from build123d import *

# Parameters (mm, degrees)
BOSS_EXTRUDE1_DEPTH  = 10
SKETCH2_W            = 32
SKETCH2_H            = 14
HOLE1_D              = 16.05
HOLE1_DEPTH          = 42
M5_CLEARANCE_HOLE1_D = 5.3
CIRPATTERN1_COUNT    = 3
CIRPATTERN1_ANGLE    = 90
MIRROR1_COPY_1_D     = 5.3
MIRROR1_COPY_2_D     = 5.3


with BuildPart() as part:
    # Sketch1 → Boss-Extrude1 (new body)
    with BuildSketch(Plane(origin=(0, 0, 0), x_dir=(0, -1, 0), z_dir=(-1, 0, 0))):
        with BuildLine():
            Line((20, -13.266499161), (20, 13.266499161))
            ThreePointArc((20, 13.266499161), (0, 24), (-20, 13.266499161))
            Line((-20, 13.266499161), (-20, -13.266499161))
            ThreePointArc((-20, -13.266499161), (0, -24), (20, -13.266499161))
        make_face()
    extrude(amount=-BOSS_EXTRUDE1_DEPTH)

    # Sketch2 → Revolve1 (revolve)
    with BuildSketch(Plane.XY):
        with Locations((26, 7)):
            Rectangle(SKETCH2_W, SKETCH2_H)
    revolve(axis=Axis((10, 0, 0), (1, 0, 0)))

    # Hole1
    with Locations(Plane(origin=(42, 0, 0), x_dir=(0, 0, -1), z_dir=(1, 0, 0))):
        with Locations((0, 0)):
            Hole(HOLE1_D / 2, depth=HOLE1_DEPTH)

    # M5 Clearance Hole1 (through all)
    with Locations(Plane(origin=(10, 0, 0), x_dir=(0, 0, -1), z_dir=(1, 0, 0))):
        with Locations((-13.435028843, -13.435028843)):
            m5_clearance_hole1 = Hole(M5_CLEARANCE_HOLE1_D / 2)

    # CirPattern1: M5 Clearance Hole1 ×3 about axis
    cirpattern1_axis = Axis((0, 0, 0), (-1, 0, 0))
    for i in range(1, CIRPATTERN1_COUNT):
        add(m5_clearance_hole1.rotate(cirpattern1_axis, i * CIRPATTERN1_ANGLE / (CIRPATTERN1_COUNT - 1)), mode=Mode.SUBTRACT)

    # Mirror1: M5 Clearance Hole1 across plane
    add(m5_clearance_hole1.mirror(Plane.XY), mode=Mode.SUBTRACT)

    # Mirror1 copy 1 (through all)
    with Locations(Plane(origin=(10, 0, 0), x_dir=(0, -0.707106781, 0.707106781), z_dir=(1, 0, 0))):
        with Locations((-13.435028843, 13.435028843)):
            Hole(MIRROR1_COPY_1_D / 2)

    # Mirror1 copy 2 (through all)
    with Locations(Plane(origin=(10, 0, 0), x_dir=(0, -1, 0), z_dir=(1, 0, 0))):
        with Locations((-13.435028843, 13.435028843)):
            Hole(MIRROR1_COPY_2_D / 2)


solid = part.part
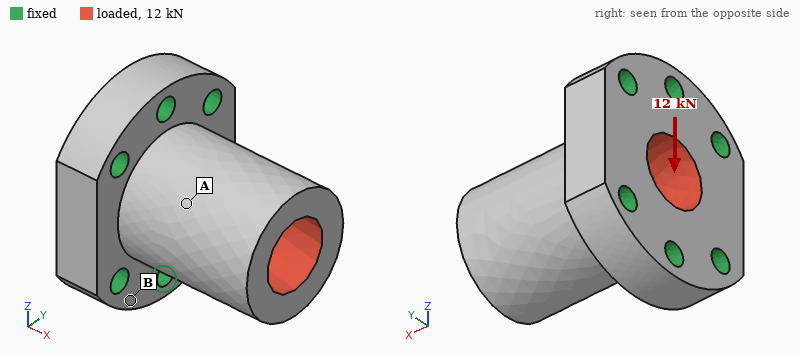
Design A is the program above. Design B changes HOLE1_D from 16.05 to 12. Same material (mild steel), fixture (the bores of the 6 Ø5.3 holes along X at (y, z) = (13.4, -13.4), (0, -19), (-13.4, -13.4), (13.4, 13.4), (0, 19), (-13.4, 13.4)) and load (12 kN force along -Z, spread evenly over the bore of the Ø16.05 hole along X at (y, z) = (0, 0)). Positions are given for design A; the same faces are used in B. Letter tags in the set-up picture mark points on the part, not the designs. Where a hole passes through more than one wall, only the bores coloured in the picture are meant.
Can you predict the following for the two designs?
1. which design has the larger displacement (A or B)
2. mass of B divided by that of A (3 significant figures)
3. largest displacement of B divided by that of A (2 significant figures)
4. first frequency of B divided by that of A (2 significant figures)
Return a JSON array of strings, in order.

["A", "1.14", "0.87", "0.97"]
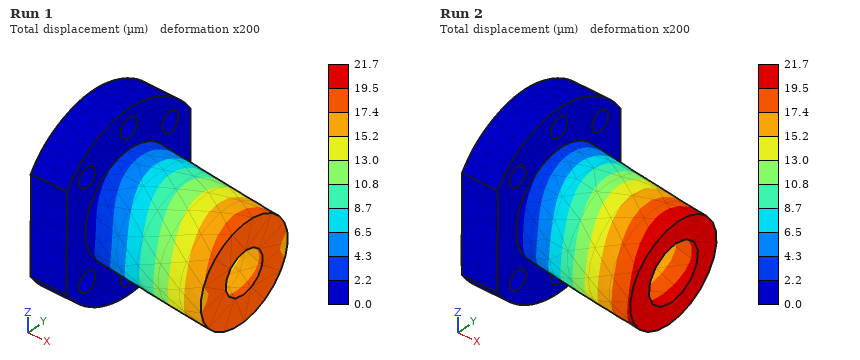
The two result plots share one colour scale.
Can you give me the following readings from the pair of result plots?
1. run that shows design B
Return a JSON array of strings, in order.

["Run 1"]
